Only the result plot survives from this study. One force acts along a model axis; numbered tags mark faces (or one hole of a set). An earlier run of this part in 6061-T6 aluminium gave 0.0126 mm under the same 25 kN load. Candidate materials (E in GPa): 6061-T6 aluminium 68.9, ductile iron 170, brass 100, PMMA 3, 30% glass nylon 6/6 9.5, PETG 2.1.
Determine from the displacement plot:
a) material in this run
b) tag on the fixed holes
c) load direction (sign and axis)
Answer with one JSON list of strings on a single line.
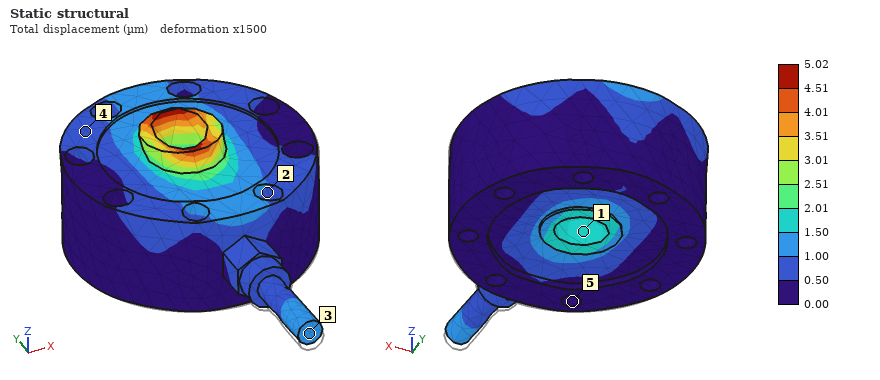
["ductile iron", "5", "+Y"]
